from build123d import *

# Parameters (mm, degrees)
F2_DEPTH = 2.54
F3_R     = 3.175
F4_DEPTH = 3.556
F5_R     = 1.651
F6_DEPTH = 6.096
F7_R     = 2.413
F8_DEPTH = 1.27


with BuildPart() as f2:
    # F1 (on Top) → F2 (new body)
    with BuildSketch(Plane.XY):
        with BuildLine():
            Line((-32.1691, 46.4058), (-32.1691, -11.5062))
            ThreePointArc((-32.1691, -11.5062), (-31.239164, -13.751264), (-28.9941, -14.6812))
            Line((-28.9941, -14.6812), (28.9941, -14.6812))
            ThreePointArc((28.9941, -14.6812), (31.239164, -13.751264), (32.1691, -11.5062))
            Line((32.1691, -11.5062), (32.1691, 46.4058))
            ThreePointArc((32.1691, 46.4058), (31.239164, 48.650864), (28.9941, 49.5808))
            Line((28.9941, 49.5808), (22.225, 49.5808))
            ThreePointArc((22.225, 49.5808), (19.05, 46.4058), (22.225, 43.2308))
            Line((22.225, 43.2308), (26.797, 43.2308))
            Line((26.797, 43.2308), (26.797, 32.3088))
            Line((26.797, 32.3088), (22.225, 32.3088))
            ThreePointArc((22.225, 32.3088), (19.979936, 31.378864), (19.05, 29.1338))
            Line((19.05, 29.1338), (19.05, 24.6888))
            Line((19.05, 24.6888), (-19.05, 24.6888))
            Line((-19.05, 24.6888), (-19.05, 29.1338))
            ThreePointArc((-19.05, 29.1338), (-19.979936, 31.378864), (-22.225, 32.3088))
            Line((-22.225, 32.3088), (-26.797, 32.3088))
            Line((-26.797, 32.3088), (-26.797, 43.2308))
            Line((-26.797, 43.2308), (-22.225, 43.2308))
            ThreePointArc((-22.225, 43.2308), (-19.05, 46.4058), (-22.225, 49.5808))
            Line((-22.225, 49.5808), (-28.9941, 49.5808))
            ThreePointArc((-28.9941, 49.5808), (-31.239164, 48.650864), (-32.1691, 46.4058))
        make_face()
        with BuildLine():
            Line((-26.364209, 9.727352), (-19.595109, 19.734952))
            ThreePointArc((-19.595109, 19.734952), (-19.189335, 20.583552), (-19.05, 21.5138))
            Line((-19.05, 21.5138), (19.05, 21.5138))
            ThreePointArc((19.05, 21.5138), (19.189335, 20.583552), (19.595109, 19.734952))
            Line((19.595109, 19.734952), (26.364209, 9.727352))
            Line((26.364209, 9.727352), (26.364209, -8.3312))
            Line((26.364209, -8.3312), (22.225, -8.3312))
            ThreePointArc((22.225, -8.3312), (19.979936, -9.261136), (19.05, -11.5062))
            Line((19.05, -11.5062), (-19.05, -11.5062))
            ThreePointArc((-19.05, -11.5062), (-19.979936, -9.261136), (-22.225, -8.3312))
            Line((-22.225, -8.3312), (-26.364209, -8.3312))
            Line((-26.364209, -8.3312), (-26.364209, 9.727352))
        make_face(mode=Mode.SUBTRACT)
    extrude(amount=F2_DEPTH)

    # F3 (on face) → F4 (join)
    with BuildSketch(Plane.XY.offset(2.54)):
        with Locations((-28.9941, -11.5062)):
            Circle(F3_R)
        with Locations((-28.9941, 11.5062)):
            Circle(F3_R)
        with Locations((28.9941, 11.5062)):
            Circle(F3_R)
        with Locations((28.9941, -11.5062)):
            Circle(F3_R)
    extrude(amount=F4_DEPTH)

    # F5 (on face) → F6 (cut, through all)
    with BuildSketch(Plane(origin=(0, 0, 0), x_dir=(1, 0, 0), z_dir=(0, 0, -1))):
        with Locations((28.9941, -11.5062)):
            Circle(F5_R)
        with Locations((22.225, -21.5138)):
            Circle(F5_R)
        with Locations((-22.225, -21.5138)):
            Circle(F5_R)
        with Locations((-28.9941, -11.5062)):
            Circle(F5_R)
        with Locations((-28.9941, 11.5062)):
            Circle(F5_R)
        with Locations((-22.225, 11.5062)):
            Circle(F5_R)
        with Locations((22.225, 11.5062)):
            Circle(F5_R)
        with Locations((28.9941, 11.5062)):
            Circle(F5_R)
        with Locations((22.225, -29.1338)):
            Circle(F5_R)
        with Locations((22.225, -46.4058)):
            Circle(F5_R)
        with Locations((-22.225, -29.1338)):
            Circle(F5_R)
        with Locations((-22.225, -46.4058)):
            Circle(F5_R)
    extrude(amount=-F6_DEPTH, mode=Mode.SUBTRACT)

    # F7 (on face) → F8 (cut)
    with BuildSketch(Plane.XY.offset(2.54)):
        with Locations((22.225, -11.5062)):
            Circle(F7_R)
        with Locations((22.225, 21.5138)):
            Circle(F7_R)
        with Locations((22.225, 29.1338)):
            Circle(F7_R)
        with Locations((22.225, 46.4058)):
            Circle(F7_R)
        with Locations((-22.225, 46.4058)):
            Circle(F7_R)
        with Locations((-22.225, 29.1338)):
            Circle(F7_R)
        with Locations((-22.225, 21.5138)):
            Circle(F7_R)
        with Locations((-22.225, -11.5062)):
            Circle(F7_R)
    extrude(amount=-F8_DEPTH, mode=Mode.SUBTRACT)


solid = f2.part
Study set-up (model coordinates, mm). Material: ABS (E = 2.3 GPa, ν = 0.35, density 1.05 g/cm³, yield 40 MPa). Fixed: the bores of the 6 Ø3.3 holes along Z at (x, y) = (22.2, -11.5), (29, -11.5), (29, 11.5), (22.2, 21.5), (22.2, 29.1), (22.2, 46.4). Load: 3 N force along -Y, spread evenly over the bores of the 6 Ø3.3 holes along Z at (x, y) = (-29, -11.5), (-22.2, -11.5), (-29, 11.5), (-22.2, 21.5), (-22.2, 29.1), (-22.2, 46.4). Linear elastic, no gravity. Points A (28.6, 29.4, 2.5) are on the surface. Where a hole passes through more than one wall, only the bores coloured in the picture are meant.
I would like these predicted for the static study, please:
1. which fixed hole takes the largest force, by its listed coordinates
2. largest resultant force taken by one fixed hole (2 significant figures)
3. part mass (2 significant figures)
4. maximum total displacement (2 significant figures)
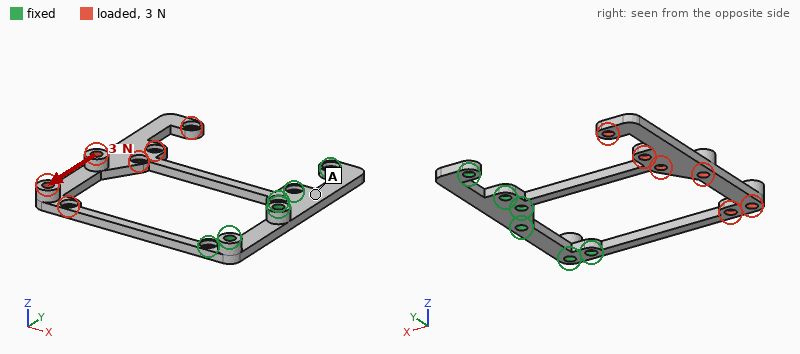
(22.2, 29.1)
5.0 N
3.7 g
0.73 mm
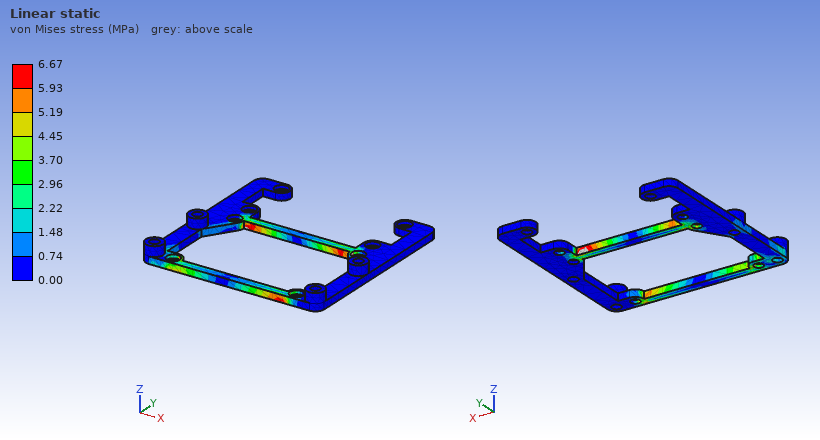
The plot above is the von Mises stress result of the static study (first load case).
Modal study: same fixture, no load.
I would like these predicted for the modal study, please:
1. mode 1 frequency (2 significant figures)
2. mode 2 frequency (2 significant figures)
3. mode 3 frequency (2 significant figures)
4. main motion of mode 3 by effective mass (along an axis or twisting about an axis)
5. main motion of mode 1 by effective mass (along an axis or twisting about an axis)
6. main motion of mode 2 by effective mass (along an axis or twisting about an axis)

83 Hz
190 Hz
260 Hz
along Y
along Z
twisting about X
